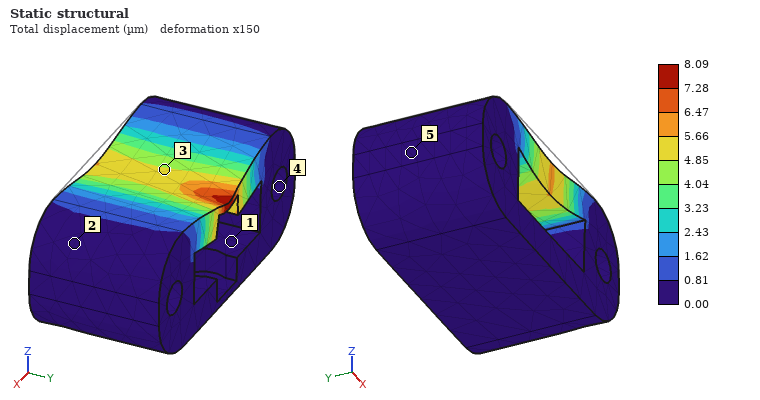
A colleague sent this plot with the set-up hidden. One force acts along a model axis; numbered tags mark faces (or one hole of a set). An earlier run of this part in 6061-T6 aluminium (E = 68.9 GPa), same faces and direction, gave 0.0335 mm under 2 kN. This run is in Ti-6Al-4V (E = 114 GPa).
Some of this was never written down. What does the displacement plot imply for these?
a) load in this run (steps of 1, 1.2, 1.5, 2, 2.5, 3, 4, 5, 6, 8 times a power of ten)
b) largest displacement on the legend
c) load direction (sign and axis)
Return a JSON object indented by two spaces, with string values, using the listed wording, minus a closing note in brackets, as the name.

{
  "load in this run": "800 N",
  "largest displacement on the legend": "8.09 µm",
  "load direction": "-Z"
}
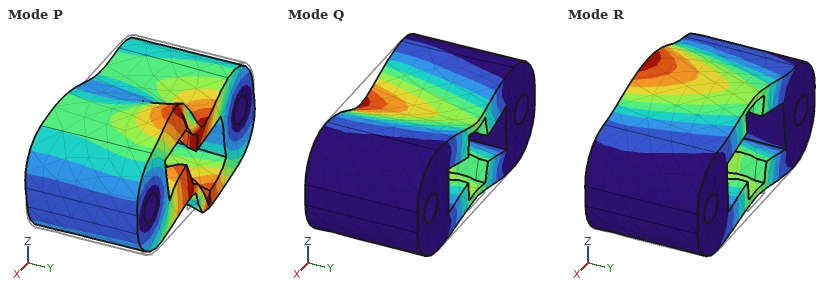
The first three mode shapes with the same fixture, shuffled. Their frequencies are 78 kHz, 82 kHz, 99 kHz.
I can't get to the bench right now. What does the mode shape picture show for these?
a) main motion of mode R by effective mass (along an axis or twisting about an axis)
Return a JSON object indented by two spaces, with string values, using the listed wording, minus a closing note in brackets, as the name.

{
  "main motion of mode R by effective mass": "along Z"
}
